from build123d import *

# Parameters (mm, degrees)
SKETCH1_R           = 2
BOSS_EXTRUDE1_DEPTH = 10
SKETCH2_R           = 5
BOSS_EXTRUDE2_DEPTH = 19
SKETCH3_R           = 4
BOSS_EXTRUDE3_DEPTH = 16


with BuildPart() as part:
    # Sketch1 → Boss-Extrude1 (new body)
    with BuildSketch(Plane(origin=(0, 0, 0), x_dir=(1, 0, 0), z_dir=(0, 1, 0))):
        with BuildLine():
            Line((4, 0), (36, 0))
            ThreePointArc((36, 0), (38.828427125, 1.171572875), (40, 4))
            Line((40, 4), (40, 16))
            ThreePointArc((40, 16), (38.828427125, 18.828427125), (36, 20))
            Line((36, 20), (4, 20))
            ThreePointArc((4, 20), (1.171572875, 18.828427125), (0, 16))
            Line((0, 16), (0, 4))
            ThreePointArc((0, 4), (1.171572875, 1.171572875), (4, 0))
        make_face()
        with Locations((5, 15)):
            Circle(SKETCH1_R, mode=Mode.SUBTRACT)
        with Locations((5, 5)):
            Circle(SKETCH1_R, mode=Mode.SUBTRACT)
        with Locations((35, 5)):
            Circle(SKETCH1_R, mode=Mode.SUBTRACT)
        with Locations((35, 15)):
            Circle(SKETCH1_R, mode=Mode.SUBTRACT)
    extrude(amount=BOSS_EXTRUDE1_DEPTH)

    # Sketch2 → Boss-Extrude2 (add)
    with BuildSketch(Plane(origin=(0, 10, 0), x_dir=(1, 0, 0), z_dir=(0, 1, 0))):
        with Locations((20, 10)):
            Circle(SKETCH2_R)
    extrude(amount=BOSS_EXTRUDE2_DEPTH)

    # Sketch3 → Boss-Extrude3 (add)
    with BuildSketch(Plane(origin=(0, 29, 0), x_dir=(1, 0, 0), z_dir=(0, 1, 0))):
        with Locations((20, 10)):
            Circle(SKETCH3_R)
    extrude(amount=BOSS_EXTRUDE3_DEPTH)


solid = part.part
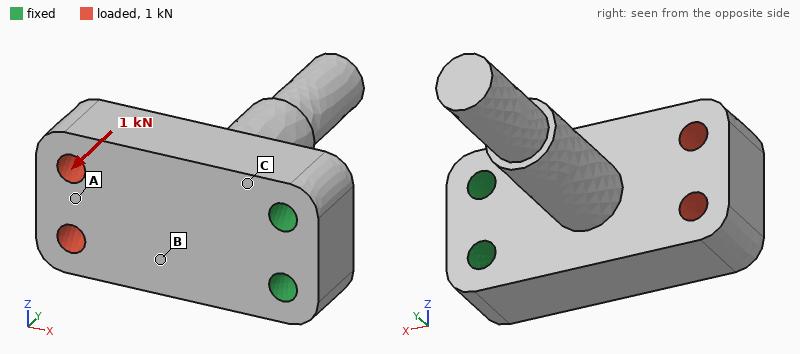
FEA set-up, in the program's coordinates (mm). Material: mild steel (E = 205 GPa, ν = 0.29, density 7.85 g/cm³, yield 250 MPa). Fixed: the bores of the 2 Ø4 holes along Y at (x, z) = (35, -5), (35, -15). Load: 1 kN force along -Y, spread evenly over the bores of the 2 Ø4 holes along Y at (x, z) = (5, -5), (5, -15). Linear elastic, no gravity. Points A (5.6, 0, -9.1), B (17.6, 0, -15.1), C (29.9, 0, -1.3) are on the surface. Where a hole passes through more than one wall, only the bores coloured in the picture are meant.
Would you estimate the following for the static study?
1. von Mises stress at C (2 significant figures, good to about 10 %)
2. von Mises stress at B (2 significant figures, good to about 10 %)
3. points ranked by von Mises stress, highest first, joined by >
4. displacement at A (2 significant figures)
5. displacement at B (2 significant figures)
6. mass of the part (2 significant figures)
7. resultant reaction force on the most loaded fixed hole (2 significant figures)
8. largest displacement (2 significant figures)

65 MPa
35 MPa
C > B > A
26 µm
12 µm
76 g
500 N
40 µm
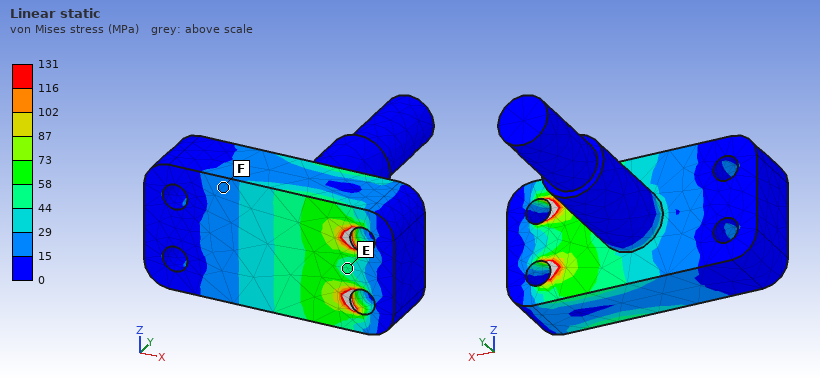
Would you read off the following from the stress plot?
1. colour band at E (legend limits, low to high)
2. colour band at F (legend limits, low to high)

44 to 58 MPa
15 to 29 MPa
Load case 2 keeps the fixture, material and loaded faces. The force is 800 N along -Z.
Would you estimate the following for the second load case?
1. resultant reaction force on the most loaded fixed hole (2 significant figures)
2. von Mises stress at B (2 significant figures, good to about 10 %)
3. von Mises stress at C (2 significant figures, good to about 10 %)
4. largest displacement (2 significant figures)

1.9 kN
12 MPa
21 MPa
9.0 µm
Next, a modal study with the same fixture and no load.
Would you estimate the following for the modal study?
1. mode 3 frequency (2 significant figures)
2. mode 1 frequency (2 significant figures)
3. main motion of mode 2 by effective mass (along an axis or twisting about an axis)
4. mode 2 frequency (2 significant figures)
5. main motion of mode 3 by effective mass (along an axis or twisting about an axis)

8800 Hz
4400 Hz
along Z
5100 Hz
along Y
